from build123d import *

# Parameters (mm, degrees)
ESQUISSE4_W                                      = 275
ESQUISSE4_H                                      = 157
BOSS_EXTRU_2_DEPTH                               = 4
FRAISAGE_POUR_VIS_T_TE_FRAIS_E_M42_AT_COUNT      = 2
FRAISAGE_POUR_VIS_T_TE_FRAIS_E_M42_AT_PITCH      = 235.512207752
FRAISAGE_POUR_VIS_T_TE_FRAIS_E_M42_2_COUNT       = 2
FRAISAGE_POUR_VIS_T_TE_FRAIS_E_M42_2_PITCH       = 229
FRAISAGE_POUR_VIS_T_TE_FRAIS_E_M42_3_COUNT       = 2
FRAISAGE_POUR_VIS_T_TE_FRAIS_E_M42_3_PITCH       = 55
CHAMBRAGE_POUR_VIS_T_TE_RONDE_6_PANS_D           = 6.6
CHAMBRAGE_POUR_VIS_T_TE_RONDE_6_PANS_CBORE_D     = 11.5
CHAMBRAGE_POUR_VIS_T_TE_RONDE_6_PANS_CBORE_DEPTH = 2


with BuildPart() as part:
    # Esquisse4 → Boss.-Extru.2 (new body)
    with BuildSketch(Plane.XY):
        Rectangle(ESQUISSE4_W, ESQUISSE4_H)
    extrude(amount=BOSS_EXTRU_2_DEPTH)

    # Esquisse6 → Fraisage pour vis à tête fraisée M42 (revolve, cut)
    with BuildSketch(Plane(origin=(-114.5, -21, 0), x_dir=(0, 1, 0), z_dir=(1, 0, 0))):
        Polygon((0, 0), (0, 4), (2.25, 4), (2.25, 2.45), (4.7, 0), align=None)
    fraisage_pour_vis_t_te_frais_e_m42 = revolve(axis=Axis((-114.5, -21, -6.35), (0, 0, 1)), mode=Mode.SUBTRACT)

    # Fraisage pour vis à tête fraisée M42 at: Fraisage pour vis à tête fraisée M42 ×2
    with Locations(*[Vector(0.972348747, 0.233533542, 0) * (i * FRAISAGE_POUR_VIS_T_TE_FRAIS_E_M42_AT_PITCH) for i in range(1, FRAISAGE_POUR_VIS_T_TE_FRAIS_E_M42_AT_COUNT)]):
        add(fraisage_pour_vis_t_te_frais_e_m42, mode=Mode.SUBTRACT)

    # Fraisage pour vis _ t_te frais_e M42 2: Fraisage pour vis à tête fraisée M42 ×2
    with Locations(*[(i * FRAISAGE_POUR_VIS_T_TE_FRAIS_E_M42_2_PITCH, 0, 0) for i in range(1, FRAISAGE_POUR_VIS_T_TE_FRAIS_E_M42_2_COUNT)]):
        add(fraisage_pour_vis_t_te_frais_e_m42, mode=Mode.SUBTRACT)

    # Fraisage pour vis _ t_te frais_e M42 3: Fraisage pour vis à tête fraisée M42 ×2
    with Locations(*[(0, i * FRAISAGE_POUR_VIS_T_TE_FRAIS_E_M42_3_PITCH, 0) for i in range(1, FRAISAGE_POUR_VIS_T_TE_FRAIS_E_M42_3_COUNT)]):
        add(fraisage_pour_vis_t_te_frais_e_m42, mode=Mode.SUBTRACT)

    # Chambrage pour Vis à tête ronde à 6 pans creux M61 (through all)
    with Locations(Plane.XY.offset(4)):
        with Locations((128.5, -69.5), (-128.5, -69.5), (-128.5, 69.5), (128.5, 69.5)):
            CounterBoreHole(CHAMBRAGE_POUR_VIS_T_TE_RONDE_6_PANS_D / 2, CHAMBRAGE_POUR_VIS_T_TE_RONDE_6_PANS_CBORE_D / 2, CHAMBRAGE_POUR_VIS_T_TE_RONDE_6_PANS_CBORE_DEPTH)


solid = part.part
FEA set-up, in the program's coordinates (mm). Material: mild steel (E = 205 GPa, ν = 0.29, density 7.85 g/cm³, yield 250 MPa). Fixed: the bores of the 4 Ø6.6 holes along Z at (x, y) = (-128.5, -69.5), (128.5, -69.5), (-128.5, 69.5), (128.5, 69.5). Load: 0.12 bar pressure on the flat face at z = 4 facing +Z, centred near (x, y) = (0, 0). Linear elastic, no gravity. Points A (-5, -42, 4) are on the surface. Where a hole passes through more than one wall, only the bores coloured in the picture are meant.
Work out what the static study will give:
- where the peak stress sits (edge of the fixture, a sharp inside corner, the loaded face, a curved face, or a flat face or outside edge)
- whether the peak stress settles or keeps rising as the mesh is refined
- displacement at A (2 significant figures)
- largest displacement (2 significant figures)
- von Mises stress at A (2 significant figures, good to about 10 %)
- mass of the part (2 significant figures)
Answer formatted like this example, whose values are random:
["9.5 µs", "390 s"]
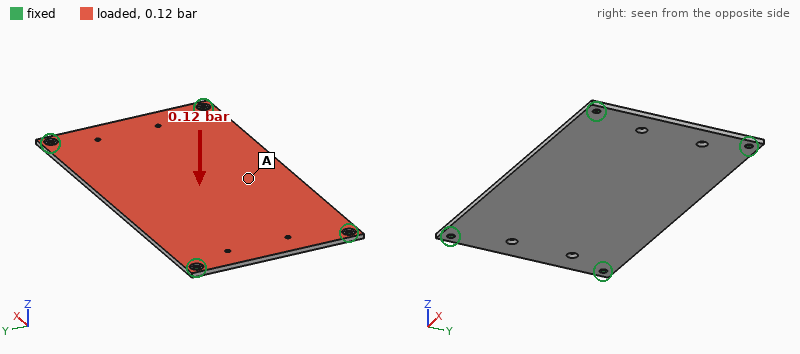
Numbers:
["edge of the fixture", "keeps rising", "0.23 mm", "0.23 mm", "17 MPa", "1.3 kg"]
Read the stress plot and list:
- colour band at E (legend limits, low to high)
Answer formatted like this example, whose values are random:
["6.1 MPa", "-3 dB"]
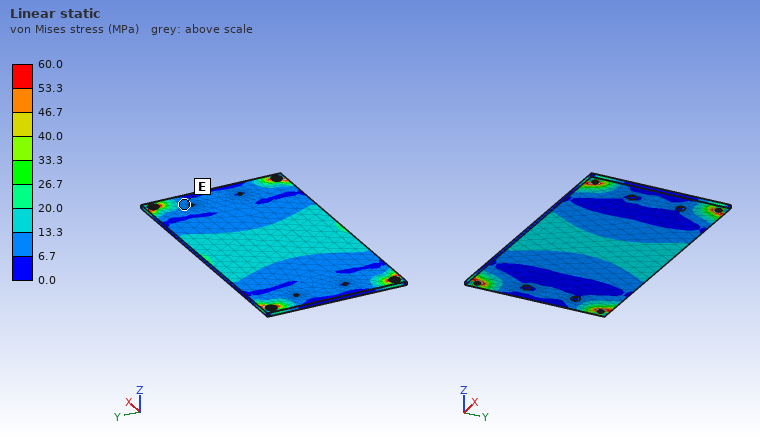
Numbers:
["6.7 to 13.3 MPa"]
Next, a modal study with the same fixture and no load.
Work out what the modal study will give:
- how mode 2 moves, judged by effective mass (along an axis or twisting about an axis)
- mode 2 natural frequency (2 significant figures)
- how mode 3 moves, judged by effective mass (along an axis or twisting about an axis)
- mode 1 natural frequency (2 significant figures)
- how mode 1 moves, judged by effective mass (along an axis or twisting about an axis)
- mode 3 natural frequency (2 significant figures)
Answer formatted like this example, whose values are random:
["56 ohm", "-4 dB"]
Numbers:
["twisting about X", "440 Hz", "twisting about Y", "230 Hz", "along Z", "640 Hz"]
